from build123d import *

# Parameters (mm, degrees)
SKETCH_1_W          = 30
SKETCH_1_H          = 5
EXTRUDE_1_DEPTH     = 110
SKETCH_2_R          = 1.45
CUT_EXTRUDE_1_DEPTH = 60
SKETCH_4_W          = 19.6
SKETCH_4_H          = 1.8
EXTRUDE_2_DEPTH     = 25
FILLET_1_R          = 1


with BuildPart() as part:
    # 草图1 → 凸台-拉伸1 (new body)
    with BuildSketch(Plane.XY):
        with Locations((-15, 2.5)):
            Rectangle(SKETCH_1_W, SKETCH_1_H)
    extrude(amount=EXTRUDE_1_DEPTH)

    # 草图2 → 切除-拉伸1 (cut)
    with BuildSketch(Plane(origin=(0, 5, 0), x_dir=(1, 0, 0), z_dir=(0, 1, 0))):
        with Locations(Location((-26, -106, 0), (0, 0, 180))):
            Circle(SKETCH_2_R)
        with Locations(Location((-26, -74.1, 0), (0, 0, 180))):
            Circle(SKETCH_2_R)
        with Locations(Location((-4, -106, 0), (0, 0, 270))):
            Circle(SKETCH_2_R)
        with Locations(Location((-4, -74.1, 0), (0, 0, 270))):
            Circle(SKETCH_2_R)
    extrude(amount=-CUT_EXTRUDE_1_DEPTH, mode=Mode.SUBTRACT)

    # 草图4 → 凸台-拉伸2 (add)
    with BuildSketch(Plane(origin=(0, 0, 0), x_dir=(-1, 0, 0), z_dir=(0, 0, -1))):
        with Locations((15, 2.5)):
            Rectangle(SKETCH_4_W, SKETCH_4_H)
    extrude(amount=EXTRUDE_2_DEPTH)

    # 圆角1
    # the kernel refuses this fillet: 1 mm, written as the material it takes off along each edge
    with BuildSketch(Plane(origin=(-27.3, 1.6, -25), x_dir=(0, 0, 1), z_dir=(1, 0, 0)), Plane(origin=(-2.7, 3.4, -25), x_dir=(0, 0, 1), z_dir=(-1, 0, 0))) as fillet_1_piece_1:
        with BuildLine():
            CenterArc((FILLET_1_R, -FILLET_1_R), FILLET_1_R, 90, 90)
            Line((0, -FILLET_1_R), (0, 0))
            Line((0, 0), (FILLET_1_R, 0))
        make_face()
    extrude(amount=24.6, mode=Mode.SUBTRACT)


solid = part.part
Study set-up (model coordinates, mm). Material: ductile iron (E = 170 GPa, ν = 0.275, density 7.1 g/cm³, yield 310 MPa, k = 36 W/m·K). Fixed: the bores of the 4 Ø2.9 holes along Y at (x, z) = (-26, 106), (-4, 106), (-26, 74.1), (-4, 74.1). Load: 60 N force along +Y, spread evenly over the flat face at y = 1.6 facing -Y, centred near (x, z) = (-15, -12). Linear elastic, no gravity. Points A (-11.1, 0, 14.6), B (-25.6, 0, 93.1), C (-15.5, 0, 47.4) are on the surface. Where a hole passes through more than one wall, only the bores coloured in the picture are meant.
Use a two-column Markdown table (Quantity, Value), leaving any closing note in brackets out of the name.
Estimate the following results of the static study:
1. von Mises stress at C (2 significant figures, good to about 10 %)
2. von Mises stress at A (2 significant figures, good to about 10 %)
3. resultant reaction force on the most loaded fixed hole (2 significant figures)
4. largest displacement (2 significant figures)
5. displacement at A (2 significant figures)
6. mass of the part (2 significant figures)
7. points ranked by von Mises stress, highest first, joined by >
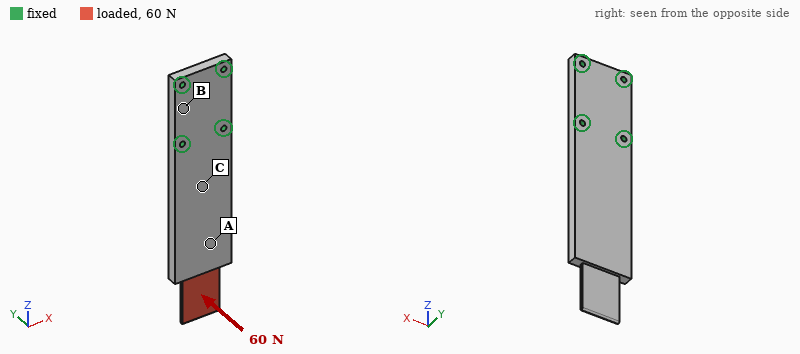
| Quantity | Value |
|---|---|
| von Mises stress at C | 28 MPa |
| von Mises stress at A | 13 MPa |
| resultant reaction force on the most loaded fixed hole | 50 N |
| largest displacement | 0.37 mm |
| displacement at A | 0.14 mm |
| mass of the part | 120 g |
| points ranked by von Mises stress, highest first, joined by > | C > A > B |
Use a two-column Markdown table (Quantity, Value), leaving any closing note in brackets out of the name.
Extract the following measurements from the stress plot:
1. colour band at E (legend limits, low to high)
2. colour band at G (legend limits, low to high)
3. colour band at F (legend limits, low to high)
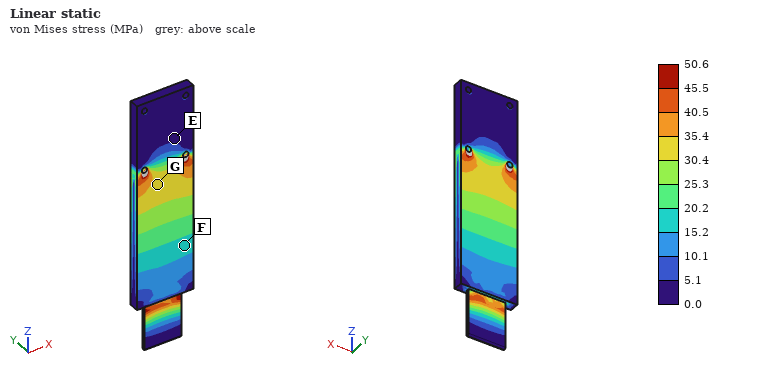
| Quantity | Value |
|---|---|
| colour band at E | 0.0 to 5.1 MPa |
| colour band at G | 30.4 to 35.4 MPa |
| colour band at F | 15.2 to 20.2 MPa |
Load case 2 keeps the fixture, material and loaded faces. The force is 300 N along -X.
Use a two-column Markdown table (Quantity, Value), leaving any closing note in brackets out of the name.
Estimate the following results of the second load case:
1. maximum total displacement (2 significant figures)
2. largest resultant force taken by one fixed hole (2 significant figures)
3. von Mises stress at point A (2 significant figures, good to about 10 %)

| Quantity | Value |
|---|---|
| maximum total displacement | 52 µm |
| largest resultant force taken by one fixed hole | 1.1 kN |
| von Mises stress at point A | 7.6 MPa |
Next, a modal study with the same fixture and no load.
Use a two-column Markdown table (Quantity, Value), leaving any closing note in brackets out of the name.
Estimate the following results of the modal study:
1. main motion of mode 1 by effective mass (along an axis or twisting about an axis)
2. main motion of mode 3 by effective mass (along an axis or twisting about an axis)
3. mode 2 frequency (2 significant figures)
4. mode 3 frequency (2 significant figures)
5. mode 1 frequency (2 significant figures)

| Quantity | Value |
|---|---|
| main motion of mode 1 by effective mass | along Y |
| main motion of mode 3 by effective mass | along X |
| mode 2 frequency | 2200 Hz |
| mode 3 frequency | 3200 Hz |
| mode 1 frequency | 570 Hz |
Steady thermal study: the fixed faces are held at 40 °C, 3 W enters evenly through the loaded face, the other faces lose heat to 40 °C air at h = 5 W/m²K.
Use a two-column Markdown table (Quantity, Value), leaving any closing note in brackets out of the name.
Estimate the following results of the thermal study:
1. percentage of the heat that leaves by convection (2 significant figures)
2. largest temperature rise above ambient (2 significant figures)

| Quantity | Value |
|---|---|
| percentage of the heat that leaves by convection | 22 % |
| largest temperature rise above ambient | 63 K |
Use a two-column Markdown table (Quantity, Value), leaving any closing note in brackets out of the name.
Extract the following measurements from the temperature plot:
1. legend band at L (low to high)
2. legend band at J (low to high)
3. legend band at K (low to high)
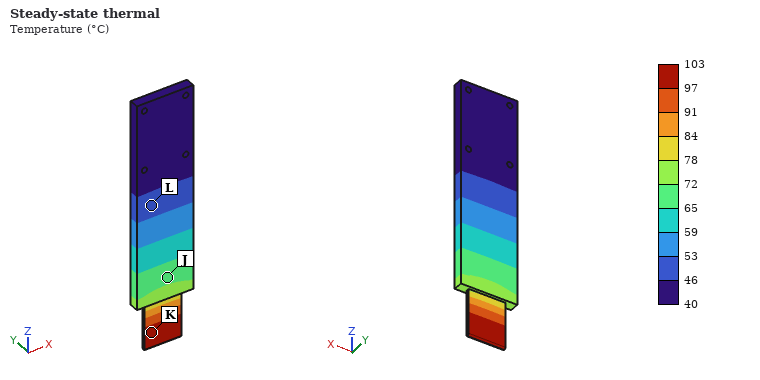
| Quantity | Value |
|---|---|
| legend band at L | 46 to 53 °C |
| legend band at J | 65 to 72 °C |
| legend band at K | 97 to 103 °C |
